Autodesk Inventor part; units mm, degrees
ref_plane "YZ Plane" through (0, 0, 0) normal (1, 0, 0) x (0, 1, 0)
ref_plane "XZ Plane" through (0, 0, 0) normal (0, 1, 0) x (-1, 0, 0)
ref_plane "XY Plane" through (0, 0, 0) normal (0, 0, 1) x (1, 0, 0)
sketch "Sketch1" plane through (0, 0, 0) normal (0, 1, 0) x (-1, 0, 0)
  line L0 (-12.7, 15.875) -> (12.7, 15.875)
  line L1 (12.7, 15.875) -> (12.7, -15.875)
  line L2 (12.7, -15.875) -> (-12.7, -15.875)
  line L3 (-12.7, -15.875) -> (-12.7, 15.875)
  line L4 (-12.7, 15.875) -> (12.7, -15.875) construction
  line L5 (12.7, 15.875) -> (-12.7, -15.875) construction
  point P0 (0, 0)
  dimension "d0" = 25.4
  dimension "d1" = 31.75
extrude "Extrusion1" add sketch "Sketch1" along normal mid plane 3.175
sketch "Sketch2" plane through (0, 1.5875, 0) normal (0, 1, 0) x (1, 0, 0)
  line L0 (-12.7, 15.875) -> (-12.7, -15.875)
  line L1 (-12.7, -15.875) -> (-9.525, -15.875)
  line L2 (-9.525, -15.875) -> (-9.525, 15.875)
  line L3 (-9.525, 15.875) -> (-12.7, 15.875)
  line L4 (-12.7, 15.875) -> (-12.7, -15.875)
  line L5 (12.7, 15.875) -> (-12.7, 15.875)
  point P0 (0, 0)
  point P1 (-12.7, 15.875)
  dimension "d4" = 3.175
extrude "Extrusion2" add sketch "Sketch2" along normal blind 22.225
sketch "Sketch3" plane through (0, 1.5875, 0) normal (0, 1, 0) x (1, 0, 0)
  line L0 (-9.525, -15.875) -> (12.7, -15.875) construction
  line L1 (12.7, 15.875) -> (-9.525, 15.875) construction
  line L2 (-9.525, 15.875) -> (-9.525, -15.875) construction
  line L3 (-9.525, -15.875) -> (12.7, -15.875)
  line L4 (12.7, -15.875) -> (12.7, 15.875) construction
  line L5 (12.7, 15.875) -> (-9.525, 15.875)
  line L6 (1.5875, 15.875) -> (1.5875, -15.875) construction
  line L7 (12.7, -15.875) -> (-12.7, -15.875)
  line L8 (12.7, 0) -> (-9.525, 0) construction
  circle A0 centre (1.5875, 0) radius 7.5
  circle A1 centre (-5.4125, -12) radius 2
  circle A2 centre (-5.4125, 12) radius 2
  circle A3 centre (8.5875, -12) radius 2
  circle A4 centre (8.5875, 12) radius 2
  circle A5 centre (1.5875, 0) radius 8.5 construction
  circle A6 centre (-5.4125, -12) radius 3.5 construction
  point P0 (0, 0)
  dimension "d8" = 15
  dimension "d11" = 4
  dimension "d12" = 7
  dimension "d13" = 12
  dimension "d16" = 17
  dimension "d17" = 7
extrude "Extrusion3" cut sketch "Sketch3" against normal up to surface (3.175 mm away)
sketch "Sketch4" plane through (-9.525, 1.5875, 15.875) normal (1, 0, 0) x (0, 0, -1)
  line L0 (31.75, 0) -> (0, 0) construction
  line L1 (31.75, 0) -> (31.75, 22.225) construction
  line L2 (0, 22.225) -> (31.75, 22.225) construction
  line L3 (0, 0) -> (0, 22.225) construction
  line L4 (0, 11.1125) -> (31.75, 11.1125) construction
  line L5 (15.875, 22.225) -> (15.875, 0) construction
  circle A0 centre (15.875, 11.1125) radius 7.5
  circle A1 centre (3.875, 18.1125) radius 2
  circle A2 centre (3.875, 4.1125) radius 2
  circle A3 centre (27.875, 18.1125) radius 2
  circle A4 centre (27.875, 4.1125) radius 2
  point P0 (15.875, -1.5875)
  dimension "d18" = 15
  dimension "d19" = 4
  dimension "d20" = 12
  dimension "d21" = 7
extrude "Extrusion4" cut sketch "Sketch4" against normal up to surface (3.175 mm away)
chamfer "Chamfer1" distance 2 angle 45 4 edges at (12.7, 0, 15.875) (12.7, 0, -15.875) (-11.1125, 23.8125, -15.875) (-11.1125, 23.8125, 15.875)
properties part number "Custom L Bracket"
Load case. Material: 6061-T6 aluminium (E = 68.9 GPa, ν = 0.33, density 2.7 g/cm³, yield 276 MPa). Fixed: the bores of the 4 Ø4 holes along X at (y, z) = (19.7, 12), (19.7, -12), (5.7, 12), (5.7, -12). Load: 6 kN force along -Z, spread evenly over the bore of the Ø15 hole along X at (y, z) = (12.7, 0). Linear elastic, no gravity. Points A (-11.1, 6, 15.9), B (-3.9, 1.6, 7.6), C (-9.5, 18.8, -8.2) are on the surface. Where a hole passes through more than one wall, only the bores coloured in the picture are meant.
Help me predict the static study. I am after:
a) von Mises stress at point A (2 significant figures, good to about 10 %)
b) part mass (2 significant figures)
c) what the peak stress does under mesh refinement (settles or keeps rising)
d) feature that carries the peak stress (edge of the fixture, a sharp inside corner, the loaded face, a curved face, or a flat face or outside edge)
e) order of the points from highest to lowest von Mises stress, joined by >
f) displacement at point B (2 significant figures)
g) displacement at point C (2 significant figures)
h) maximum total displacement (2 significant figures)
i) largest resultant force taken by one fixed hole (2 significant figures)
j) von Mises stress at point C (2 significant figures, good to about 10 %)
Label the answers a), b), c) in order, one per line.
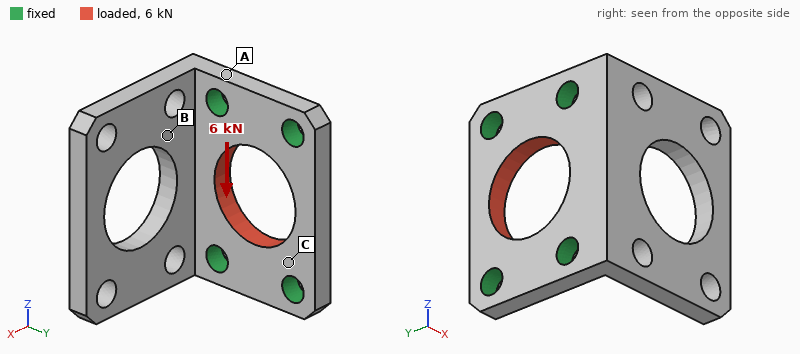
a) 27 MPa
b) 9.0 g
c) keeps rising
d) edge of the fixture
e) C > A > B
f) 2.4 µm
g) 1.9 µm
h) 7.2 µm
i) 1.5 kN
j) 62 MPa
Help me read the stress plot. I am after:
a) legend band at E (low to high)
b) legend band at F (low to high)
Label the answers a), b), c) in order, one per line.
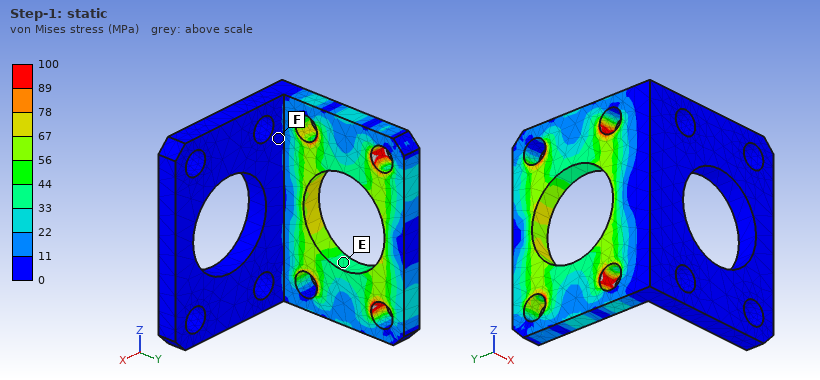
a) 33 to 44 MPa
b) 0 to 11 MPa
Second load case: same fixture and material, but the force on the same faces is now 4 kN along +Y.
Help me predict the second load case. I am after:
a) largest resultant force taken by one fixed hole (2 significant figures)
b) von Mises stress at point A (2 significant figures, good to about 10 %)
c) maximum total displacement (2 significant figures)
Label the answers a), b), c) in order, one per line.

a) 1.1 kN
b) 14 MPa
c) 20 µm
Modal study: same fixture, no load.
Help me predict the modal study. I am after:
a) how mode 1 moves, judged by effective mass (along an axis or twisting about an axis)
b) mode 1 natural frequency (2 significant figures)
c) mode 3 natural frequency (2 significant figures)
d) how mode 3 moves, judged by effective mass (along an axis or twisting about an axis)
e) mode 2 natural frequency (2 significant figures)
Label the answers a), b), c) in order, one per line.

a) along Y
b) 3400 Hz
c) 13 kHz
d) along Z
e) 6800 Hz
